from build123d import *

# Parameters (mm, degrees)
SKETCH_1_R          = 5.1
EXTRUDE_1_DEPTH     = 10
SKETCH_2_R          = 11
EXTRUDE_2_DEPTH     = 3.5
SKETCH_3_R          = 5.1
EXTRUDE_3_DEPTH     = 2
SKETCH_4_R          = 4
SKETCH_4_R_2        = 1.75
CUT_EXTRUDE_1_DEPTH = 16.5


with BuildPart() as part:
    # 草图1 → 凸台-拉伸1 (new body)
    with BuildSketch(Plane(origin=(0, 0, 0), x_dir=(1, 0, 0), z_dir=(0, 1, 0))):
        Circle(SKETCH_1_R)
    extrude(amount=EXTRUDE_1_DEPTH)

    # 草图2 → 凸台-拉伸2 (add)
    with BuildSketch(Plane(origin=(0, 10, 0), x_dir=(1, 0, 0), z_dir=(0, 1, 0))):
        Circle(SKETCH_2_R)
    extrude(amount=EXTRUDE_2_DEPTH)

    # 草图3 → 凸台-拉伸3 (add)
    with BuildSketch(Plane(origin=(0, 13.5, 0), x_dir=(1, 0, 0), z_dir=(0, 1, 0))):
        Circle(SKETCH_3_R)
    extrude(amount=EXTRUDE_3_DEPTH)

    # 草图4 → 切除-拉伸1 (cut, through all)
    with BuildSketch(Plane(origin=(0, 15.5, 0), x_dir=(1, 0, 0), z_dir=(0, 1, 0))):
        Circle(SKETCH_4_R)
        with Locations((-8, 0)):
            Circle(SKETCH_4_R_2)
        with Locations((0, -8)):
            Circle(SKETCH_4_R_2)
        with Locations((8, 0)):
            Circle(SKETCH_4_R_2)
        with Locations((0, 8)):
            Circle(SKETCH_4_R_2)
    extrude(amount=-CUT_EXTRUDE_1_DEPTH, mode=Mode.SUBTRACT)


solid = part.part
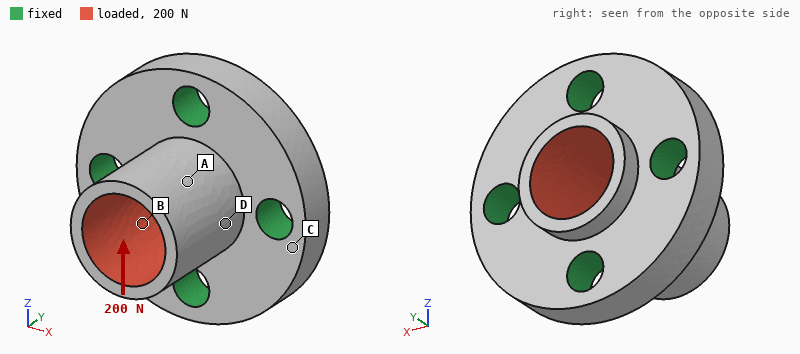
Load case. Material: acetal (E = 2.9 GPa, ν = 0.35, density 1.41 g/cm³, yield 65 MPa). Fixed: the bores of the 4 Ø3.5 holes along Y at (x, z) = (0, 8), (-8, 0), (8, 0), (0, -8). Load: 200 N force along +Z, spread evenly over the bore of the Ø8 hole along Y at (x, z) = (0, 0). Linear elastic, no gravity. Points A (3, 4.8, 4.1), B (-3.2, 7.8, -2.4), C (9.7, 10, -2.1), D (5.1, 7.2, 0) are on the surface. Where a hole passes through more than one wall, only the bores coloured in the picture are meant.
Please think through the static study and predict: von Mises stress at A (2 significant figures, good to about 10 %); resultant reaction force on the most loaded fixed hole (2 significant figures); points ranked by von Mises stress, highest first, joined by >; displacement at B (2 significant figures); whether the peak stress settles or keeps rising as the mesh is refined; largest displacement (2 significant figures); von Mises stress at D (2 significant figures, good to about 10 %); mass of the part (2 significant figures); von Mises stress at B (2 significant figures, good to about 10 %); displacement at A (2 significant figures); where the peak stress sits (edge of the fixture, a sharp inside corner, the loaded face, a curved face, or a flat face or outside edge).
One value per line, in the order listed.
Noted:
4.3 MPa
81 N
B > D > A > C
24 µm
keeps rising
80 µm
8.0 MPa
2.0 g
11 MPa
51 µm
a sharp inside corner
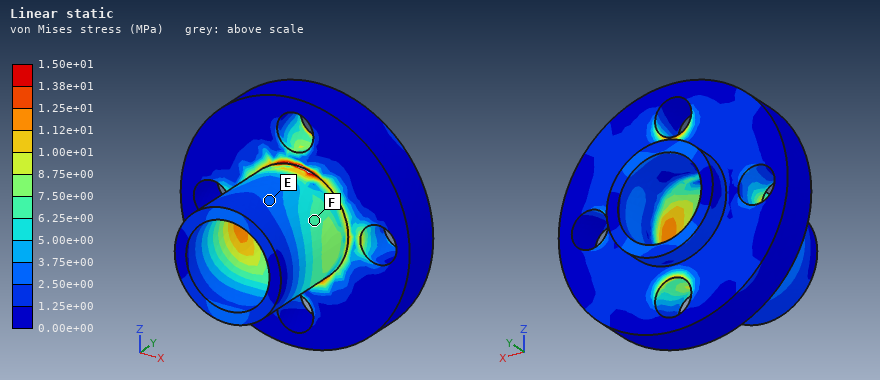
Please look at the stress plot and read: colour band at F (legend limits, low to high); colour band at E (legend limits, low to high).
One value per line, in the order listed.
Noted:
6.25e+00 to 7.50e+00 MPa
2.50e+00 to 3.75e+00 MPa
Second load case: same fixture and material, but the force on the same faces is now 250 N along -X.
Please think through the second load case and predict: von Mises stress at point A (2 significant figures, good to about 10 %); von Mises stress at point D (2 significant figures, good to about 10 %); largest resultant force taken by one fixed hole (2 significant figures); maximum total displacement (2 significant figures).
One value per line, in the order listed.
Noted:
6.7 MPa
4.5 MPa
100 N
100 µm
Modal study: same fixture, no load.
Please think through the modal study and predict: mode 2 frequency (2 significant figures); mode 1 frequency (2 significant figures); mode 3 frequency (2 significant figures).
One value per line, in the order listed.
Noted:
11 kHz
11 kHz
12 kHz
